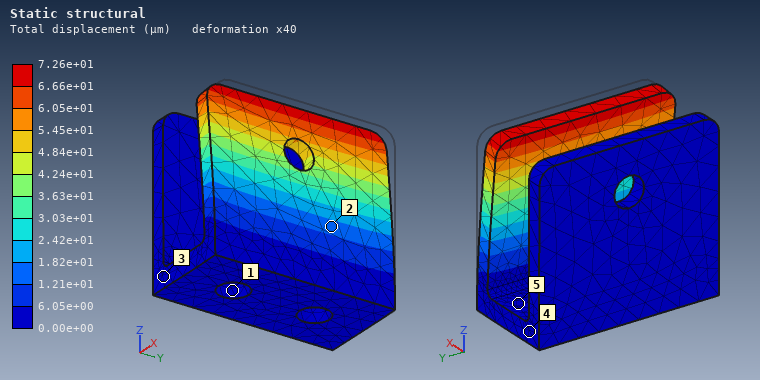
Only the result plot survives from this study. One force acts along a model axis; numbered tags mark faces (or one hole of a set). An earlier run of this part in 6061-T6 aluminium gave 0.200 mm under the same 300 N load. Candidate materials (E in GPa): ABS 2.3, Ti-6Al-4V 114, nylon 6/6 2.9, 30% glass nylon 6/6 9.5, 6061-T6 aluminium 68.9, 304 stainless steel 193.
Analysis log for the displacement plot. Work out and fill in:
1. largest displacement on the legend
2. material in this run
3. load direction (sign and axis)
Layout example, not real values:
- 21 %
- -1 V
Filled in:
- 7.26e+01 µm
- 304 stainless steel
- -X
